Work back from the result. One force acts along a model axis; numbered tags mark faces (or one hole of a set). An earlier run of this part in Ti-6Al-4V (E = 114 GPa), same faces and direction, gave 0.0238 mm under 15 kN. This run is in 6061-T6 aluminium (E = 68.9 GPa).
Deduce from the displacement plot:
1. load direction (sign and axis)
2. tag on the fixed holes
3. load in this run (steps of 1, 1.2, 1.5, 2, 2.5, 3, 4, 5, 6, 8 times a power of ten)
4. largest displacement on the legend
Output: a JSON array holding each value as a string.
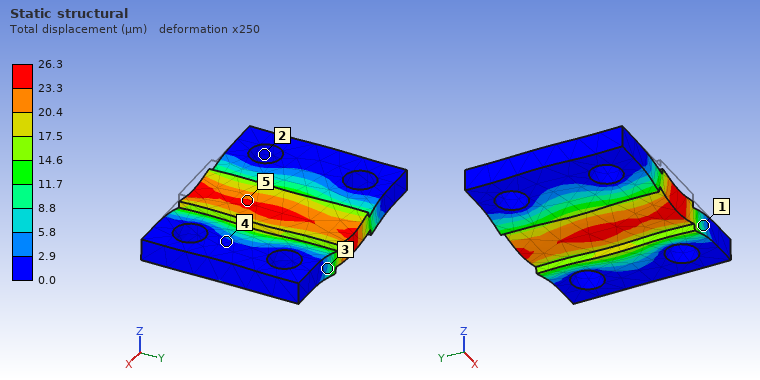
["-Z", "2", "10 kN", "26.3 µm"]
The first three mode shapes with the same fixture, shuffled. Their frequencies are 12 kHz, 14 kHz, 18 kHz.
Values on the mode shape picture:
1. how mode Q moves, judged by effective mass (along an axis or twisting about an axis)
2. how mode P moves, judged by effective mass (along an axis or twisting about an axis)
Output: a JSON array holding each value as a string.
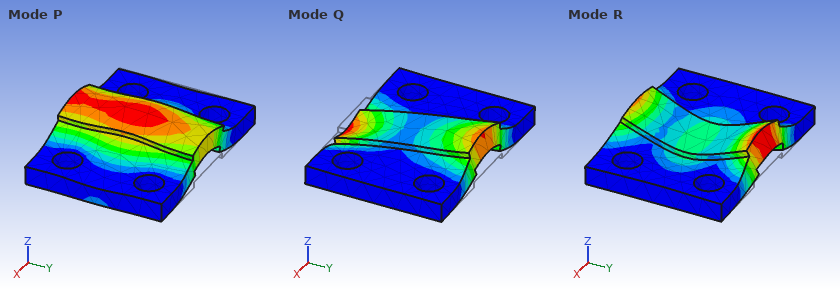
["twisting about X", "along Z"]
